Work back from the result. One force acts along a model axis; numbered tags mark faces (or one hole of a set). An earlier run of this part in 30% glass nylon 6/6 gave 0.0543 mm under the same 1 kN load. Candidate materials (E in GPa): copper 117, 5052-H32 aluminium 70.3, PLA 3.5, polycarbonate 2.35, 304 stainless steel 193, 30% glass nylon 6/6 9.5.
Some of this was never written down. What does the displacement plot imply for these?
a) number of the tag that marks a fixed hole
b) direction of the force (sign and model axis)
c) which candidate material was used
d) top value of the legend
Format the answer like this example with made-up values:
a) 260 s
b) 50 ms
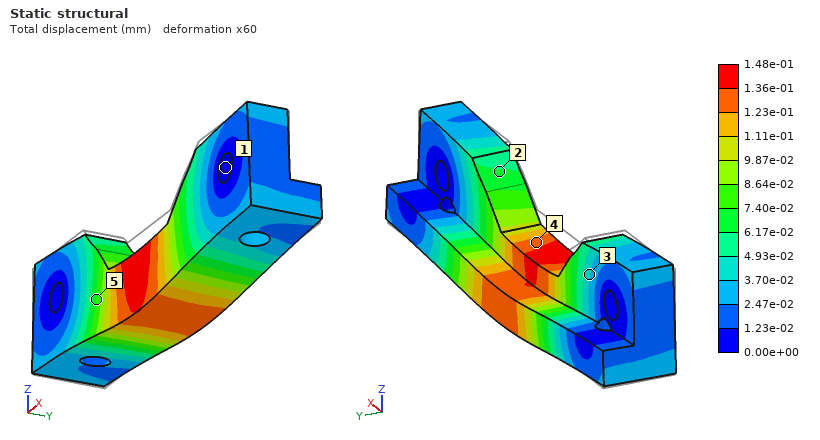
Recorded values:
a) 1
b) -Z
c) PLA
d) 1.48e-01 mm
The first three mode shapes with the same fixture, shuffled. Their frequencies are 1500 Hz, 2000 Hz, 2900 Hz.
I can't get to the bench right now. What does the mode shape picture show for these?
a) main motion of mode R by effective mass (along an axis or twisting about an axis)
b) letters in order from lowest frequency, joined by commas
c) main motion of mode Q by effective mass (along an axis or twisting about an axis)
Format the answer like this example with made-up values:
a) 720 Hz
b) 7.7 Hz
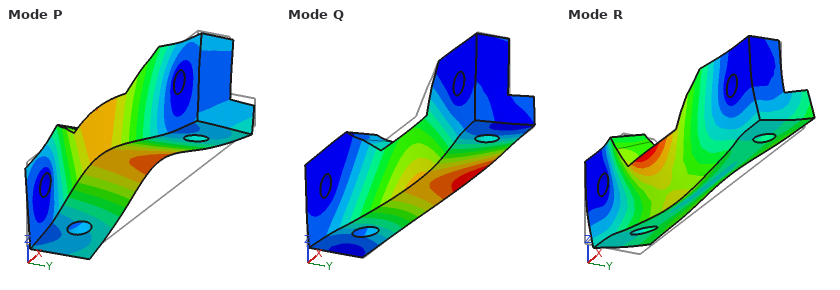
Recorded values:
a) twisting about X
b) Q, P, R
c) along Y
